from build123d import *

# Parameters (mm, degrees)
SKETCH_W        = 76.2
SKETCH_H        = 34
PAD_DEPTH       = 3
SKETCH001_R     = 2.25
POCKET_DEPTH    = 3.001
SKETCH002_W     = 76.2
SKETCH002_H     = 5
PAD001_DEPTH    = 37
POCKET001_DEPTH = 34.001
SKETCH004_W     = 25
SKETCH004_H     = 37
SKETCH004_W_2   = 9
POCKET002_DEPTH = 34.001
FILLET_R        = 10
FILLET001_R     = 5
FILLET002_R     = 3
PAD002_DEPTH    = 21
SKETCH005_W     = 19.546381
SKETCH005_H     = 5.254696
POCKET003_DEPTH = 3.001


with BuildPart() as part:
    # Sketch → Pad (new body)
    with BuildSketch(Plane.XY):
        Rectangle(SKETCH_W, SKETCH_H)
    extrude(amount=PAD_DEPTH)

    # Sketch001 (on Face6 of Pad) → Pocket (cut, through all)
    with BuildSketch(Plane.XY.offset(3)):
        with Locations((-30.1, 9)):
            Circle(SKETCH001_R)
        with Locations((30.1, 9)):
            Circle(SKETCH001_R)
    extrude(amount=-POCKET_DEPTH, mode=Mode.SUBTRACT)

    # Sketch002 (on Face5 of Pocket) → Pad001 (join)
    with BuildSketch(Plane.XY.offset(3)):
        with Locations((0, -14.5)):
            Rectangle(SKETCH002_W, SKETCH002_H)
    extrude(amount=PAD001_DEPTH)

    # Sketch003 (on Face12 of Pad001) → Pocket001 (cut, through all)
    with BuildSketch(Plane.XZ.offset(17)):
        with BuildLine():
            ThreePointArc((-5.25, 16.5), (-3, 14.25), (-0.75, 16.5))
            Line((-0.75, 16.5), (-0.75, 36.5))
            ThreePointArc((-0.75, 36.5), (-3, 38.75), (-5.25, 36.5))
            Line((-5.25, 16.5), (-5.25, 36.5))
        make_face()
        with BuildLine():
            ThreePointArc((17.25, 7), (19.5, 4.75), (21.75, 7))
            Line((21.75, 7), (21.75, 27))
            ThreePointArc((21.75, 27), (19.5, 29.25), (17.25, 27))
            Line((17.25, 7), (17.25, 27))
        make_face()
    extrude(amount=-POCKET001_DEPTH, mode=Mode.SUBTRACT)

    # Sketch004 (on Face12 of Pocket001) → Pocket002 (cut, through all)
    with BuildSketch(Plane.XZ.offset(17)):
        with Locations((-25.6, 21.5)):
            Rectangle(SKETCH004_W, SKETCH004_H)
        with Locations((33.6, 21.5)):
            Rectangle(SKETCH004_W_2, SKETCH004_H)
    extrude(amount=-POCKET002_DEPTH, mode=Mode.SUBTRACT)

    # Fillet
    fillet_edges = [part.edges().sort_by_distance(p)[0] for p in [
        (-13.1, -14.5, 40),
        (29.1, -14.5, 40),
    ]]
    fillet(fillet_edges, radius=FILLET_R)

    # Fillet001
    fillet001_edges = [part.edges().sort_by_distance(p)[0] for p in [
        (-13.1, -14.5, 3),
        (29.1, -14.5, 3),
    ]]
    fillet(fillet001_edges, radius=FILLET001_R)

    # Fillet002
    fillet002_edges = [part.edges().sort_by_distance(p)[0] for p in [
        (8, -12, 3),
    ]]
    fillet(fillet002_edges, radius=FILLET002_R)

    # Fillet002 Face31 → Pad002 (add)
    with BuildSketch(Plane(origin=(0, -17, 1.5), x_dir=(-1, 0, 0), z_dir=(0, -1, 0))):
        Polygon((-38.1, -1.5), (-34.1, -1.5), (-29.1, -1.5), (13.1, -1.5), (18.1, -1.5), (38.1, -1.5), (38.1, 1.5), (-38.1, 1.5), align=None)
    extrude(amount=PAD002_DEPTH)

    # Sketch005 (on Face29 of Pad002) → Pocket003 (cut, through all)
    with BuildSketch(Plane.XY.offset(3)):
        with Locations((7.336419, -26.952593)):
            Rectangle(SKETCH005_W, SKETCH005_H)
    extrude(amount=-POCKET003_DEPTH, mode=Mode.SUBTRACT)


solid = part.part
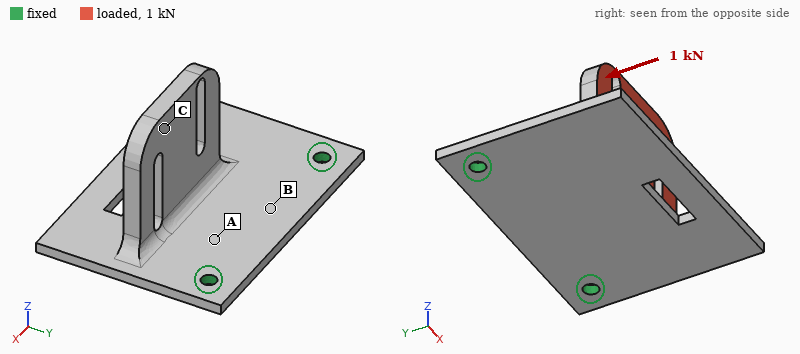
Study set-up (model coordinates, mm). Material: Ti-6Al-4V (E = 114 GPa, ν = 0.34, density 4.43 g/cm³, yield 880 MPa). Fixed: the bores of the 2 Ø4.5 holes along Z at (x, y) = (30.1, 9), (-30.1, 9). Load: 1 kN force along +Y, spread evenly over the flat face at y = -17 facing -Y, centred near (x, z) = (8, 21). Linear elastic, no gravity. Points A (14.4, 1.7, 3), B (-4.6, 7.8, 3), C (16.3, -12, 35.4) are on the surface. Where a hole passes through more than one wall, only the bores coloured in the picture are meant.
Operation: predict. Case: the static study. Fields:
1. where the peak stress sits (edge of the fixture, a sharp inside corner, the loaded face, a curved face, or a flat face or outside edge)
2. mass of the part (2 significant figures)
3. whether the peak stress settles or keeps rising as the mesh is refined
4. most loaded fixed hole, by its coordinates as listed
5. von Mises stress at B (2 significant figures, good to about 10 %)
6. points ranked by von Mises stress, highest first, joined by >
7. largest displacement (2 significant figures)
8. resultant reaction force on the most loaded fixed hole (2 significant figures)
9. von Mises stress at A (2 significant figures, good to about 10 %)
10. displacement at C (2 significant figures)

edge of the fixture
83 g
keeps rising
(30.1, 9)
66 MPa
A > B > C
1.2 mm
660 N
140 MPa
1.0 mm
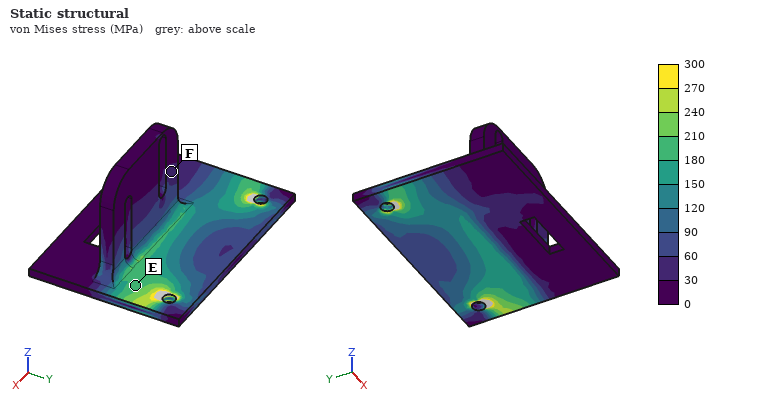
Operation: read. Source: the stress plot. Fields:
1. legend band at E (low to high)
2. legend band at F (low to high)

180 to 210 MPa
30 to 60 MPa
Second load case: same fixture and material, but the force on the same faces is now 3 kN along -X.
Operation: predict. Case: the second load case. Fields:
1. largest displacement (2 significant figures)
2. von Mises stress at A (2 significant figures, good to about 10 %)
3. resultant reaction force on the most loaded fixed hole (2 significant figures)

0.53 mm
120 MPa
2.2 kN
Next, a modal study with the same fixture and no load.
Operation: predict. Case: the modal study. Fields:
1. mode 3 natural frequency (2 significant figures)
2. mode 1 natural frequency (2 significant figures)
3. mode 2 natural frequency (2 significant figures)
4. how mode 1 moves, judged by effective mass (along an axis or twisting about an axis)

2500 Hz
700 Hz
1800 Hz
along Z
